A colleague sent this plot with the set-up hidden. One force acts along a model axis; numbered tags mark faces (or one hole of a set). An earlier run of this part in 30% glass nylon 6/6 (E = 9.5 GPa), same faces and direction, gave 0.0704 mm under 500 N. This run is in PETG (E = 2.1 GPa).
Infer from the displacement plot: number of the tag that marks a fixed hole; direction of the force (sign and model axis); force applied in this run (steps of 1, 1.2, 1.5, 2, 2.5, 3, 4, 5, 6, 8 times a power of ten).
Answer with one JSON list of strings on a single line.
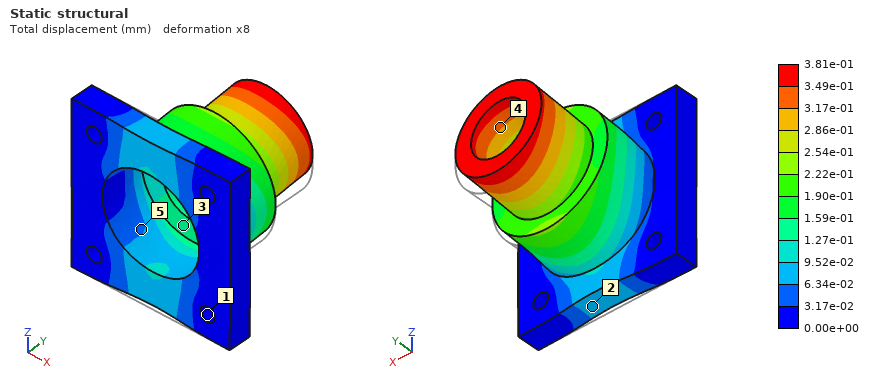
["1", "+Z", "600 N"]
